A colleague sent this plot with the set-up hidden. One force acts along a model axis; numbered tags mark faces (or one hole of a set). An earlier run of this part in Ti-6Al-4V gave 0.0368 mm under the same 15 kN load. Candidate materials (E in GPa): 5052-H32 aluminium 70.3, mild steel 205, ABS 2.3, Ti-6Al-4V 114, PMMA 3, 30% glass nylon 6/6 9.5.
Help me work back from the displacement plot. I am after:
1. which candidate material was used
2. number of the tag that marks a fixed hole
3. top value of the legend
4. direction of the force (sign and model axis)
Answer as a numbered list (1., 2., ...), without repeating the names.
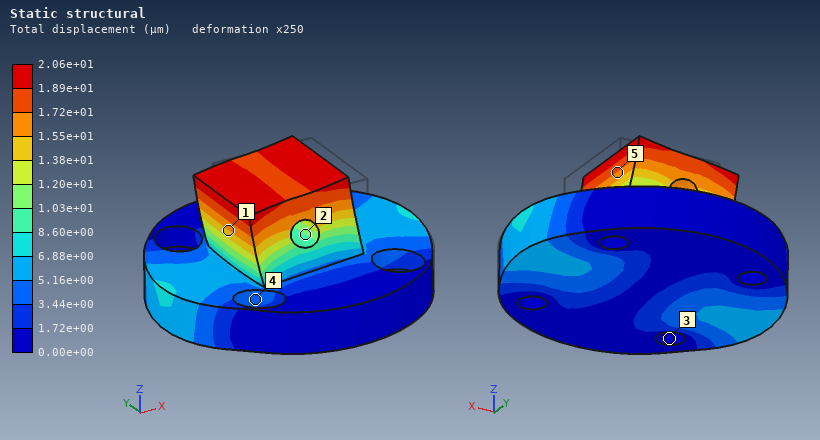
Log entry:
1. mild steel
2. 3
3. 2.06e+01 µm
4. -X
